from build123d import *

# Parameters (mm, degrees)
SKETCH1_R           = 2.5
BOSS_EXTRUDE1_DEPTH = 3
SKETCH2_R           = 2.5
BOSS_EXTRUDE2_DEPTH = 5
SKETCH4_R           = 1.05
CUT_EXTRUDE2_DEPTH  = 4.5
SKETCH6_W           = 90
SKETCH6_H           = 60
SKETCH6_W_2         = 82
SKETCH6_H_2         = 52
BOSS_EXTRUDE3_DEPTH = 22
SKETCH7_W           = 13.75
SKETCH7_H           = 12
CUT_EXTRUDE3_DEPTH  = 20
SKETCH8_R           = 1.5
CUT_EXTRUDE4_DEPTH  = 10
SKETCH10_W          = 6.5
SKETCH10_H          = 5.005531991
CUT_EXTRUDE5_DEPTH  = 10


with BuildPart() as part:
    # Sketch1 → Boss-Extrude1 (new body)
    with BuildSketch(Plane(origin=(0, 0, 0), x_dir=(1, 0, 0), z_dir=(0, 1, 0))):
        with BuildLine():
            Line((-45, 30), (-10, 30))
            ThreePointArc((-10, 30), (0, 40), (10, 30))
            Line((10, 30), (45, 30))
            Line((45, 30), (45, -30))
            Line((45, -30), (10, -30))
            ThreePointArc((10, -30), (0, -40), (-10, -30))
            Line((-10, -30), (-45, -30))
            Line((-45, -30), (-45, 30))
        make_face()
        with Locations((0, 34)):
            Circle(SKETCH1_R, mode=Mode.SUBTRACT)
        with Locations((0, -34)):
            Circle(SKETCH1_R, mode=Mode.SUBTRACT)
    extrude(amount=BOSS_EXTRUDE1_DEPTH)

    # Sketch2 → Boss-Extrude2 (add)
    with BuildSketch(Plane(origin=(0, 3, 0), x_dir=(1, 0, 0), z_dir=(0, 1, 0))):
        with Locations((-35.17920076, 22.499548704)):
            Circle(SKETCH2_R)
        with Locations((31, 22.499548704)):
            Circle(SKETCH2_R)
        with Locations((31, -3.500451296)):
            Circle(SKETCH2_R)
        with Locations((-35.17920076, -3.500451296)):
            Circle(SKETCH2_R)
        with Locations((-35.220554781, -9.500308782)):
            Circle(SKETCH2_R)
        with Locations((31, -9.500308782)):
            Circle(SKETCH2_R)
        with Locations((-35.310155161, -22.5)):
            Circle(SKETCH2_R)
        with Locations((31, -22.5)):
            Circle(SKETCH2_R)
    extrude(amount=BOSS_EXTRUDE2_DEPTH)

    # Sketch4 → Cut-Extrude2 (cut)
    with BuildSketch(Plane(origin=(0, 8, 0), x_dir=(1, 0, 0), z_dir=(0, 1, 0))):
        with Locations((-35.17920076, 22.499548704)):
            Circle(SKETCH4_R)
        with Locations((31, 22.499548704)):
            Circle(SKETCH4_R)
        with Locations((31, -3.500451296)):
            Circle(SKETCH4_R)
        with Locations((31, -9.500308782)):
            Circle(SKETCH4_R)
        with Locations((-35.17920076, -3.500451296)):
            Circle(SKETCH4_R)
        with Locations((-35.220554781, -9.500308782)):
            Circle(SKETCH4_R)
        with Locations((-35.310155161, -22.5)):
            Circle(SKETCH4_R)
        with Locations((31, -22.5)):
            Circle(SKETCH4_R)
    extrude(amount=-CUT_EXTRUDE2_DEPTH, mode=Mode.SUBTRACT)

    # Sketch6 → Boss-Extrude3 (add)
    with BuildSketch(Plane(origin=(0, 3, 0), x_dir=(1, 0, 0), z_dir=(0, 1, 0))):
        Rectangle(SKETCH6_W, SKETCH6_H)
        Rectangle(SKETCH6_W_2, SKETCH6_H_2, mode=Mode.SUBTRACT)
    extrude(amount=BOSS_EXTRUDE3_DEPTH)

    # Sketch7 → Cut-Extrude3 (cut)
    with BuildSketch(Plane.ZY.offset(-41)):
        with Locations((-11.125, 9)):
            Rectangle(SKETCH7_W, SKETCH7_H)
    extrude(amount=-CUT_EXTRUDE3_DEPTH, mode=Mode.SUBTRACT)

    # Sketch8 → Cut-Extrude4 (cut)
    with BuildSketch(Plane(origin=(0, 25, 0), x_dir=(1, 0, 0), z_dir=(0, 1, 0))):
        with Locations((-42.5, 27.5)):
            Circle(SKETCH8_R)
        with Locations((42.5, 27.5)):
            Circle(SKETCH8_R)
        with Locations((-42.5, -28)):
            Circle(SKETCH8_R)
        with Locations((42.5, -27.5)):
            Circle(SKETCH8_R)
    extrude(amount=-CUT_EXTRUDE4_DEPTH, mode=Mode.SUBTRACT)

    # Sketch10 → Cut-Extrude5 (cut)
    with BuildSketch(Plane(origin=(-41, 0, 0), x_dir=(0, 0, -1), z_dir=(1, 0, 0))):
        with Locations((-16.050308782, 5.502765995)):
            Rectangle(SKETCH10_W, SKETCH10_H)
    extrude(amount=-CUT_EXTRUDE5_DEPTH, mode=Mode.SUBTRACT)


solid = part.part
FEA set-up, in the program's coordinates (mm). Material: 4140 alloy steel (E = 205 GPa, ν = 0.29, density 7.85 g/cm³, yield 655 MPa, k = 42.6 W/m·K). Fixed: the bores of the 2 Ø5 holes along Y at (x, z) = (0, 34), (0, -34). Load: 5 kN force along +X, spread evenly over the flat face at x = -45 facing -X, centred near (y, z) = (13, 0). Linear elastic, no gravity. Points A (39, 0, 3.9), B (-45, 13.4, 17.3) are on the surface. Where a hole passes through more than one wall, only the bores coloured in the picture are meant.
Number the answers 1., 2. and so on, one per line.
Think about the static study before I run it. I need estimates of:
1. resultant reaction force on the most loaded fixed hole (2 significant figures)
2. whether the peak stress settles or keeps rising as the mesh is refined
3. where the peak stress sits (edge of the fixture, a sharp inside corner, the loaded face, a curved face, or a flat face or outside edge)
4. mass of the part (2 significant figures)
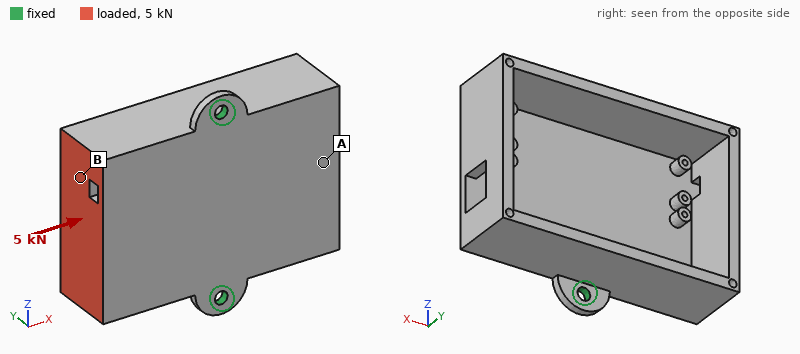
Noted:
1. 2.5 kN
2. keeps rising
3. edge of the fixture
4. 330 g
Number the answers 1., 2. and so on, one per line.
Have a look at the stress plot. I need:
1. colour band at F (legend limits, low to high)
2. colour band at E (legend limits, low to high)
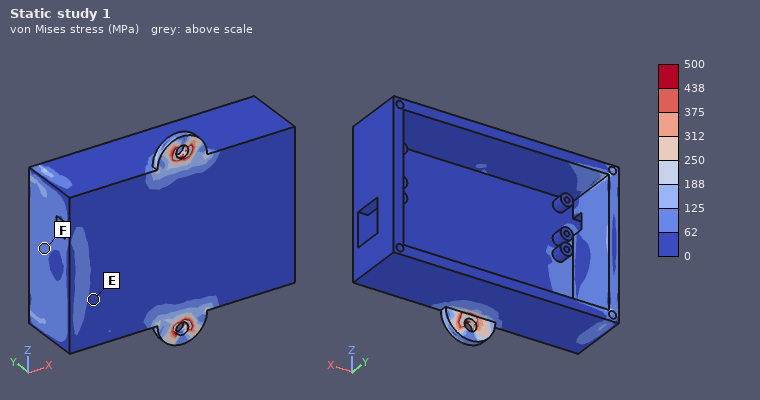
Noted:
1. 62 to 125 MPa
2. 0 to 62 MPa
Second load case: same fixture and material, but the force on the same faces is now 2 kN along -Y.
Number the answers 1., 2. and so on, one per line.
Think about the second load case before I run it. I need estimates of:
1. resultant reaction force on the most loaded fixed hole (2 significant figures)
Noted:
1. 1.0 kN
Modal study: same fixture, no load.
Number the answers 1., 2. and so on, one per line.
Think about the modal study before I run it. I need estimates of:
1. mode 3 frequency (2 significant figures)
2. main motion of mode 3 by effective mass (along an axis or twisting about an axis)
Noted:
1. 3300 Hz
2. along Y
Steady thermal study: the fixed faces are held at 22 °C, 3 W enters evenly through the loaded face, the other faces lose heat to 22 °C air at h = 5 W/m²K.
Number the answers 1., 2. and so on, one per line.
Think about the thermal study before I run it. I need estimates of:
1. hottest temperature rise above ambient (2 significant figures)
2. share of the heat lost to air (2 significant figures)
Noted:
1. 13 K
2. 21 %
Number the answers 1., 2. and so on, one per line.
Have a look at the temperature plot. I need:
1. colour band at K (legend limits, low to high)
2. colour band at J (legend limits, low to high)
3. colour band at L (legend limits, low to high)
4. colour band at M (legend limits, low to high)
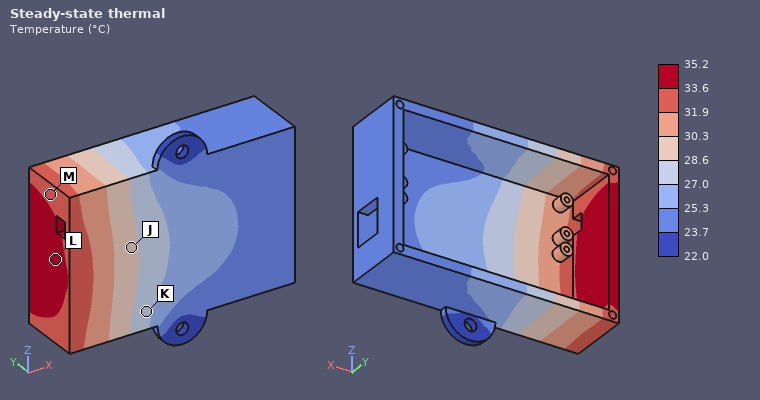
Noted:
1. 27.0 to 28.6 °C
2. 28.6 to 30.3 °C
3. 33.6 to 35.2 °C
4. 31.9 to 33.6 °C
